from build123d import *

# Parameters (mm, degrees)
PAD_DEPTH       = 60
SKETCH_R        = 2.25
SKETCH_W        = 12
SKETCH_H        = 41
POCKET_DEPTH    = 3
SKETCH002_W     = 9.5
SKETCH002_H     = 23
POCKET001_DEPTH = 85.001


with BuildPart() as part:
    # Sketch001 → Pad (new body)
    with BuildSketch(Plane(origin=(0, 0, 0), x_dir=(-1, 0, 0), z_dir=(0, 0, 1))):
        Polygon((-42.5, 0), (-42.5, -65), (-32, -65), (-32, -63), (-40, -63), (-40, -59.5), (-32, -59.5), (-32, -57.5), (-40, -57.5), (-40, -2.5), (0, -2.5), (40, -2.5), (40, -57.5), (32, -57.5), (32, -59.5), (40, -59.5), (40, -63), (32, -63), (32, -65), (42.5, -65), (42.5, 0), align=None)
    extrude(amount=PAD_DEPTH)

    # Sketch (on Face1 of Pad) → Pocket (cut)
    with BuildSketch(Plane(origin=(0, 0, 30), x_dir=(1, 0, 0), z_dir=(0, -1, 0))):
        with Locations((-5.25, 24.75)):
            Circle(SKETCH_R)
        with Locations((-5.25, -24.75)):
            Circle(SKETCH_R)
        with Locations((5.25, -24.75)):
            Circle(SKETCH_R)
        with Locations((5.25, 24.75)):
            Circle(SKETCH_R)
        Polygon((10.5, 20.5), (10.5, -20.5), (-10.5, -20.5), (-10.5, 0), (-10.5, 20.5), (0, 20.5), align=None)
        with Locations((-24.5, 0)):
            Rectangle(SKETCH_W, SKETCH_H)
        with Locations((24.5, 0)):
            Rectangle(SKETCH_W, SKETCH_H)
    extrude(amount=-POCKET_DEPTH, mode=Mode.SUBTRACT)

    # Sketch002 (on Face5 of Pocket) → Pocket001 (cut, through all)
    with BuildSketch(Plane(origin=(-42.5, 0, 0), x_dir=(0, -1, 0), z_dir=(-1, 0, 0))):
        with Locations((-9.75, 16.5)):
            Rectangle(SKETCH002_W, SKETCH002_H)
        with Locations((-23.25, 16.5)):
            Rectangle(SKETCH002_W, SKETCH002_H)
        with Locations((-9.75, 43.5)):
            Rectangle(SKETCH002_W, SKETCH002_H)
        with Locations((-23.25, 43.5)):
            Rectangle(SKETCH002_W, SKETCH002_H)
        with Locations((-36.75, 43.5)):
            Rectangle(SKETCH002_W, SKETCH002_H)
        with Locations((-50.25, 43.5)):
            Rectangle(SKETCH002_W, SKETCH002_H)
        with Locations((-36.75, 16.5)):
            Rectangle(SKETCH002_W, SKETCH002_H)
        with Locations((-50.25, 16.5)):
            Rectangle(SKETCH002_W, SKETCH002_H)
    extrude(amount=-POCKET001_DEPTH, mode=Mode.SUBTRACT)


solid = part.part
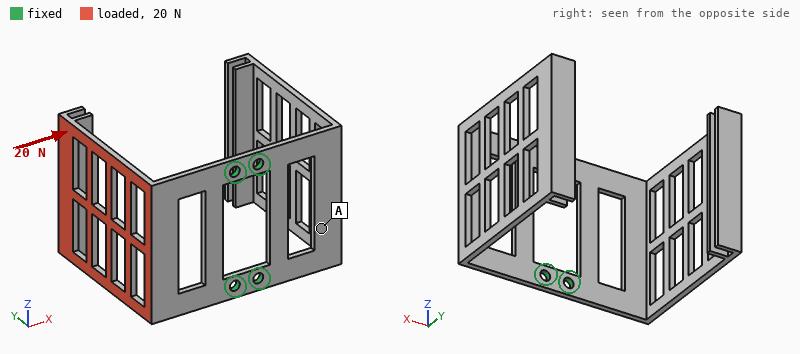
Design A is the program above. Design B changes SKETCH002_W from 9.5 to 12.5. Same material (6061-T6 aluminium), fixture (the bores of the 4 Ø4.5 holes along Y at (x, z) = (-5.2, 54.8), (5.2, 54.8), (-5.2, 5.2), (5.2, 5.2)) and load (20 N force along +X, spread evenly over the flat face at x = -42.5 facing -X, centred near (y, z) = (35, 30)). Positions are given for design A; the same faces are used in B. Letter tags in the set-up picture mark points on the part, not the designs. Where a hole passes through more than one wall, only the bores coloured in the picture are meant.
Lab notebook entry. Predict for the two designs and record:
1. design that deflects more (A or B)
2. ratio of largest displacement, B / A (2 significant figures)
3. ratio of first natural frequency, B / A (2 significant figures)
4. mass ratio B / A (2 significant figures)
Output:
B
1.1
1.0
0.87
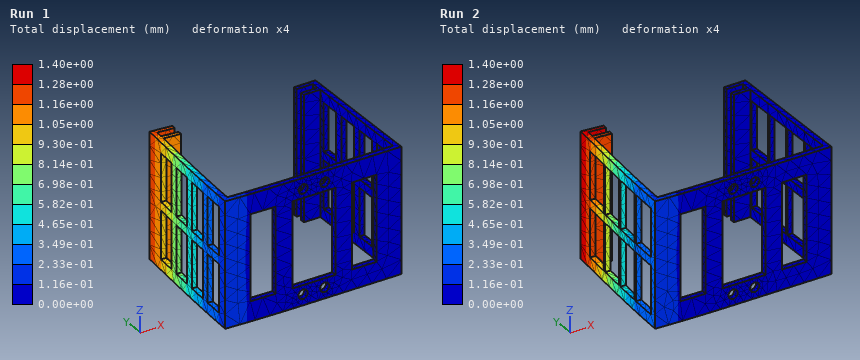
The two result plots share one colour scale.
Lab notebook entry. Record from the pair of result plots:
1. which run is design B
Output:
Run 2
